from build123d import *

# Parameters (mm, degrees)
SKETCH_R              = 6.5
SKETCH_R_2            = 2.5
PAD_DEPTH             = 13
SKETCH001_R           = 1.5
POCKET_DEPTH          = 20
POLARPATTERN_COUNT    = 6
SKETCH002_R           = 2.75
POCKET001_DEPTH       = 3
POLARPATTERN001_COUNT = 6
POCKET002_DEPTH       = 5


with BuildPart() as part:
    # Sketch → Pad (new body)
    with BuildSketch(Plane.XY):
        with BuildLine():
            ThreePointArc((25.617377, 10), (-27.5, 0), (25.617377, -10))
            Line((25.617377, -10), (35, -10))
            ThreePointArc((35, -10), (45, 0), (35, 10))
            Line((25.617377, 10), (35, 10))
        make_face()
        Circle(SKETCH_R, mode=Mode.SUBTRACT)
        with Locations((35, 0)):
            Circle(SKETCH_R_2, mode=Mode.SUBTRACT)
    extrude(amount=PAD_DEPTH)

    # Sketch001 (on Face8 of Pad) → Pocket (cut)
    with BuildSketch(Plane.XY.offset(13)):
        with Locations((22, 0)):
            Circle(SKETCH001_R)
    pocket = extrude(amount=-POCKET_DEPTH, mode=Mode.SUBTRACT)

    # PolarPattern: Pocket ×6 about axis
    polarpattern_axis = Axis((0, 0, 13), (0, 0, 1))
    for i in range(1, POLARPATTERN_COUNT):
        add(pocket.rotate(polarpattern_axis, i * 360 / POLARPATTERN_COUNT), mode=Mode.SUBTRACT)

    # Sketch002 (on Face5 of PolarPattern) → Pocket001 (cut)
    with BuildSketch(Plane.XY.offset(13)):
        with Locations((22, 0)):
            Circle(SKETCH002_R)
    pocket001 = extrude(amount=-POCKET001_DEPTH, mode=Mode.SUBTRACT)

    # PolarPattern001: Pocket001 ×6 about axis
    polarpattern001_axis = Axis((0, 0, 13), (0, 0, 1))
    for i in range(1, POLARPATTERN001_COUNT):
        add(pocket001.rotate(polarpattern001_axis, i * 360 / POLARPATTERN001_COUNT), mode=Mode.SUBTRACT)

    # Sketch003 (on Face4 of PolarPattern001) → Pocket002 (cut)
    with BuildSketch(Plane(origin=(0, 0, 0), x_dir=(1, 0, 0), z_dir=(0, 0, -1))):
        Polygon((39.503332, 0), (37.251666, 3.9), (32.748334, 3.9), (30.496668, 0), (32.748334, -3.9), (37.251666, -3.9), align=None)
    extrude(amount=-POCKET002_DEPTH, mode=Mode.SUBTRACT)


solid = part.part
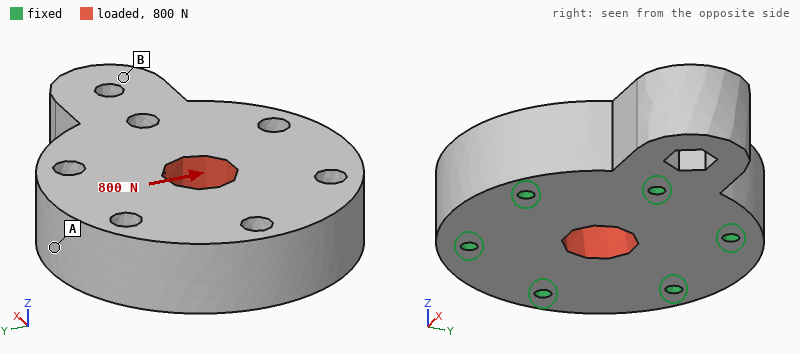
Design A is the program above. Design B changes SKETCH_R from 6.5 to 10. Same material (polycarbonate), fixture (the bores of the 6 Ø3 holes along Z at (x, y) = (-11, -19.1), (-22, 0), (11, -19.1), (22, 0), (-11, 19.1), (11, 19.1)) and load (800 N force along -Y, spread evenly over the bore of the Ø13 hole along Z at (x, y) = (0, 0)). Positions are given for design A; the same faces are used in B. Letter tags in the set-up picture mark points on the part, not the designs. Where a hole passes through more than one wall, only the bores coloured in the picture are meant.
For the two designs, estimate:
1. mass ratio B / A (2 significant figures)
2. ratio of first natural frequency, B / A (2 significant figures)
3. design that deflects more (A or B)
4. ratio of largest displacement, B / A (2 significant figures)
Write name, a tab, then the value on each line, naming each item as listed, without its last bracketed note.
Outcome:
mass ratio B / A	0.93
ratio of first natural frequency, B / A	0.99
design that deflects more	A
ratio of largest displacement, B / A	0.82
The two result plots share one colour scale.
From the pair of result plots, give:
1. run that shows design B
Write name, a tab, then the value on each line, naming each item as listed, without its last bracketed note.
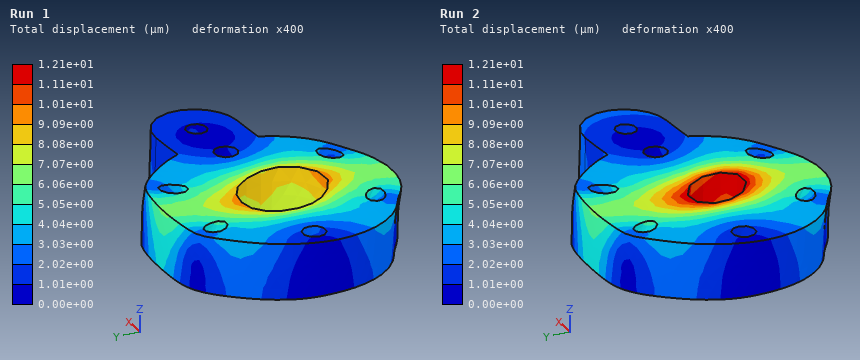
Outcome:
run that shows design B	Run 1
